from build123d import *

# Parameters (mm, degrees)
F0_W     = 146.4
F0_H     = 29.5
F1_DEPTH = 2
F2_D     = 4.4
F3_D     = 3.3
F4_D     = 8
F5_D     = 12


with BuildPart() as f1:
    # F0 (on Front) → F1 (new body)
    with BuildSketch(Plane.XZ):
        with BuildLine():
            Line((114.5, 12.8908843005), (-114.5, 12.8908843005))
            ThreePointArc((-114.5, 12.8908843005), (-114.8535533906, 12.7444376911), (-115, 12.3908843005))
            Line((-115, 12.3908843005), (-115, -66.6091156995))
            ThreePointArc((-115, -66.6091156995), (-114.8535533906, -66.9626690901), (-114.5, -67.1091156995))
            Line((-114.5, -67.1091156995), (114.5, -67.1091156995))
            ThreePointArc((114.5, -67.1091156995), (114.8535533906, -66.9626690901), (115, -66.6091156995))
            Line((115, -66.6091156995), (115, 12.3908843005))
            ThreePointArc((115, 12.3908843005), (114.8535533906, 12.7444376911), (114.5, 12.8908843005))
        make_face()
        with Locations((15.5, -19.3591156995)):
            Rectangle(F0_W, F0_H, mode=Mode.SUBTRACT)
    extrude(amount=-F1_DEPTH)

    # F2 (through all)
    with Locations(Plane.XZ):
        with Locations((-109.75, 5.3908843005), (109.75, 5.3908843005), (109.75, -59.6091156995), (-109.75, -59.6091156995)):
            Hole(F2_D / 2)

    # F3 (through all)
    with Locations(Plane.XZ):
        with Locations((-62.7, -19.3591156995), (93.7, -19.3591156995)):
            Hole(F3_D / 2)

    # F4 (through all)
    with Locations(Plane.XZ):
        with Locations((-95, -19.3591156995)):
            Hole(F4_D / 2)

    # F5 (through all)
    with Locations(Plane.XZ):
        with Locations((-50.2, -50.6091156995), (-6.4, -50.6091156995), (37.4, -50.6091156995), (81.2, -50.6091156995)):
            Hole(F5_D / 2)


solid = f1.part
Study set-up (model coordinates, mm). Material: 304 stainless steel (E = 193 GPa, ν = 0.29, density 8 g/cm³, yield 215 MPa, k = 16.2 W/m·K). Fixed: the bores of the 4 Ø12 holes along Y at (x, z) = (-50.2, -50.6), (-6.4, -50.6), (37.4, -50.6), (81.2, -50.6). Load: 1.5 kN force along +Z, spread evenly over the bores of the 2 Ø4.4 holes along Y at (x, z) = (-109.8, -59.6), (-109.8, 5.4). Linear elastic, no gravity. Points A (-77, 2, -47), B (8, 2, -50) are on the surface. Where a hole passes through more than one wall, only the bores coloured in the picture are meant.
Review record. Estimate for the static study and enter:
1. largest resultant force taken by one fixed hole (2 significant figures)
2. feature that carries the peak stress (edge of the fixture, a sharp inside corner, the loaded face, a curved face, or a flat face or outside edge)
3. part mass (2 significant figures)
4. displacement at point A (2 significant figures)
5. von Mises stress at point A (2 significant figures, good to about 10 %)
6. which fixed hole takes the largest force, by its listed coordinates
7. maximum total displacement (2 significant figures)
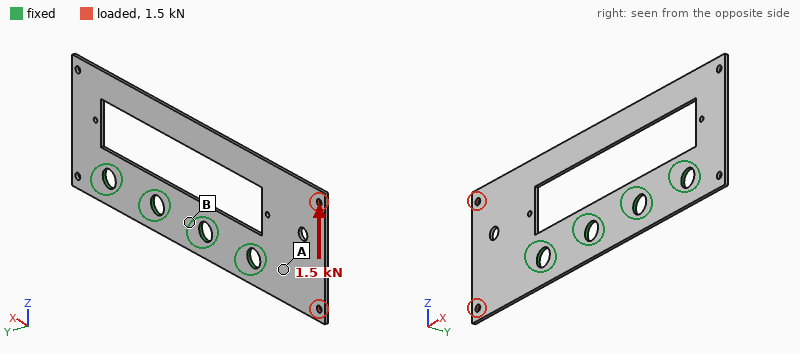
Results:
2.1 kN
edge of the fixture
220 g
0.029 mm
41 MPa
(-50.2, -50.6)
0.11 mm
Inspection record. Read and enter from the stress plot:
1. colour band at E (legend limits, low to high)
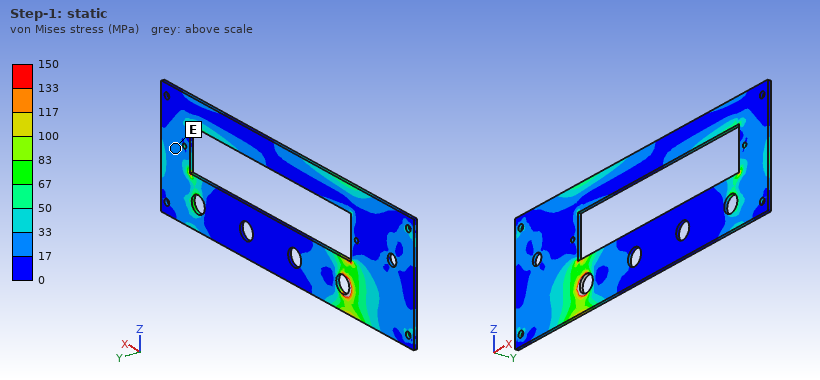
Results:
17 to 33 MPa
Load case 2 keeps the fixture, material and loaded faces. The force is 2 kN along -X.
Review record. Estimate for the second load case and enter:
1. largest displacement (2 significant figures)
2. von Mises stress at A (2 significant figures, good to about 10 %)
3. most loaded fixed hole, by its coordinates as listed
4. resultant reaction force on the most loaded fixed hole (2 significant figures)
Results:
65 µm
30 MPa
(-50.2, -50.6)
1.6 kN
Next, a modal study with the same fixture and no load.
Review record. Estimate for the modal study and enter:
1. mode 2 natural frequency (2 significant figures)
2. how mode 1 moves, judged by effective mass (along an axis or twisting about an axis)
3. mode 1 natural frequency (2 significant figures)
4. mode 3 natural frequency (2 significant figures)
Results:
250 Hz
along Y
210 Hz
390 Hz
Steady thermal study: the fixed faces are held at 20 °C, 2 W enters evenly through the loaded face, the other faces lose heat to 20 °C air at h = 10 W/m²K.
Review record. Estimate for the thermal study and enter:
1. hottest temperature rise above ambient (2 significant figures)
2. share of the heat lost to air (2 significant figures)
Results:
42 K
78 %
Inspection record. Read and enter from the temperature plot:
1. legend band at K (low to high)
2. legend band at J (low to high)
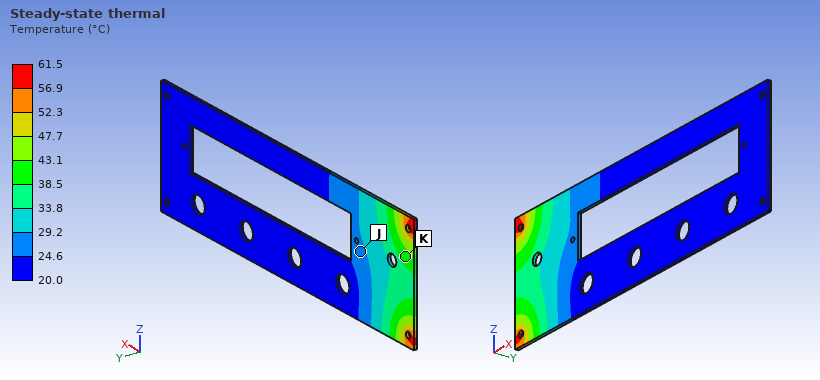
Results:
38.5 to 43.1 °C
24.6 to 29.2 °C
